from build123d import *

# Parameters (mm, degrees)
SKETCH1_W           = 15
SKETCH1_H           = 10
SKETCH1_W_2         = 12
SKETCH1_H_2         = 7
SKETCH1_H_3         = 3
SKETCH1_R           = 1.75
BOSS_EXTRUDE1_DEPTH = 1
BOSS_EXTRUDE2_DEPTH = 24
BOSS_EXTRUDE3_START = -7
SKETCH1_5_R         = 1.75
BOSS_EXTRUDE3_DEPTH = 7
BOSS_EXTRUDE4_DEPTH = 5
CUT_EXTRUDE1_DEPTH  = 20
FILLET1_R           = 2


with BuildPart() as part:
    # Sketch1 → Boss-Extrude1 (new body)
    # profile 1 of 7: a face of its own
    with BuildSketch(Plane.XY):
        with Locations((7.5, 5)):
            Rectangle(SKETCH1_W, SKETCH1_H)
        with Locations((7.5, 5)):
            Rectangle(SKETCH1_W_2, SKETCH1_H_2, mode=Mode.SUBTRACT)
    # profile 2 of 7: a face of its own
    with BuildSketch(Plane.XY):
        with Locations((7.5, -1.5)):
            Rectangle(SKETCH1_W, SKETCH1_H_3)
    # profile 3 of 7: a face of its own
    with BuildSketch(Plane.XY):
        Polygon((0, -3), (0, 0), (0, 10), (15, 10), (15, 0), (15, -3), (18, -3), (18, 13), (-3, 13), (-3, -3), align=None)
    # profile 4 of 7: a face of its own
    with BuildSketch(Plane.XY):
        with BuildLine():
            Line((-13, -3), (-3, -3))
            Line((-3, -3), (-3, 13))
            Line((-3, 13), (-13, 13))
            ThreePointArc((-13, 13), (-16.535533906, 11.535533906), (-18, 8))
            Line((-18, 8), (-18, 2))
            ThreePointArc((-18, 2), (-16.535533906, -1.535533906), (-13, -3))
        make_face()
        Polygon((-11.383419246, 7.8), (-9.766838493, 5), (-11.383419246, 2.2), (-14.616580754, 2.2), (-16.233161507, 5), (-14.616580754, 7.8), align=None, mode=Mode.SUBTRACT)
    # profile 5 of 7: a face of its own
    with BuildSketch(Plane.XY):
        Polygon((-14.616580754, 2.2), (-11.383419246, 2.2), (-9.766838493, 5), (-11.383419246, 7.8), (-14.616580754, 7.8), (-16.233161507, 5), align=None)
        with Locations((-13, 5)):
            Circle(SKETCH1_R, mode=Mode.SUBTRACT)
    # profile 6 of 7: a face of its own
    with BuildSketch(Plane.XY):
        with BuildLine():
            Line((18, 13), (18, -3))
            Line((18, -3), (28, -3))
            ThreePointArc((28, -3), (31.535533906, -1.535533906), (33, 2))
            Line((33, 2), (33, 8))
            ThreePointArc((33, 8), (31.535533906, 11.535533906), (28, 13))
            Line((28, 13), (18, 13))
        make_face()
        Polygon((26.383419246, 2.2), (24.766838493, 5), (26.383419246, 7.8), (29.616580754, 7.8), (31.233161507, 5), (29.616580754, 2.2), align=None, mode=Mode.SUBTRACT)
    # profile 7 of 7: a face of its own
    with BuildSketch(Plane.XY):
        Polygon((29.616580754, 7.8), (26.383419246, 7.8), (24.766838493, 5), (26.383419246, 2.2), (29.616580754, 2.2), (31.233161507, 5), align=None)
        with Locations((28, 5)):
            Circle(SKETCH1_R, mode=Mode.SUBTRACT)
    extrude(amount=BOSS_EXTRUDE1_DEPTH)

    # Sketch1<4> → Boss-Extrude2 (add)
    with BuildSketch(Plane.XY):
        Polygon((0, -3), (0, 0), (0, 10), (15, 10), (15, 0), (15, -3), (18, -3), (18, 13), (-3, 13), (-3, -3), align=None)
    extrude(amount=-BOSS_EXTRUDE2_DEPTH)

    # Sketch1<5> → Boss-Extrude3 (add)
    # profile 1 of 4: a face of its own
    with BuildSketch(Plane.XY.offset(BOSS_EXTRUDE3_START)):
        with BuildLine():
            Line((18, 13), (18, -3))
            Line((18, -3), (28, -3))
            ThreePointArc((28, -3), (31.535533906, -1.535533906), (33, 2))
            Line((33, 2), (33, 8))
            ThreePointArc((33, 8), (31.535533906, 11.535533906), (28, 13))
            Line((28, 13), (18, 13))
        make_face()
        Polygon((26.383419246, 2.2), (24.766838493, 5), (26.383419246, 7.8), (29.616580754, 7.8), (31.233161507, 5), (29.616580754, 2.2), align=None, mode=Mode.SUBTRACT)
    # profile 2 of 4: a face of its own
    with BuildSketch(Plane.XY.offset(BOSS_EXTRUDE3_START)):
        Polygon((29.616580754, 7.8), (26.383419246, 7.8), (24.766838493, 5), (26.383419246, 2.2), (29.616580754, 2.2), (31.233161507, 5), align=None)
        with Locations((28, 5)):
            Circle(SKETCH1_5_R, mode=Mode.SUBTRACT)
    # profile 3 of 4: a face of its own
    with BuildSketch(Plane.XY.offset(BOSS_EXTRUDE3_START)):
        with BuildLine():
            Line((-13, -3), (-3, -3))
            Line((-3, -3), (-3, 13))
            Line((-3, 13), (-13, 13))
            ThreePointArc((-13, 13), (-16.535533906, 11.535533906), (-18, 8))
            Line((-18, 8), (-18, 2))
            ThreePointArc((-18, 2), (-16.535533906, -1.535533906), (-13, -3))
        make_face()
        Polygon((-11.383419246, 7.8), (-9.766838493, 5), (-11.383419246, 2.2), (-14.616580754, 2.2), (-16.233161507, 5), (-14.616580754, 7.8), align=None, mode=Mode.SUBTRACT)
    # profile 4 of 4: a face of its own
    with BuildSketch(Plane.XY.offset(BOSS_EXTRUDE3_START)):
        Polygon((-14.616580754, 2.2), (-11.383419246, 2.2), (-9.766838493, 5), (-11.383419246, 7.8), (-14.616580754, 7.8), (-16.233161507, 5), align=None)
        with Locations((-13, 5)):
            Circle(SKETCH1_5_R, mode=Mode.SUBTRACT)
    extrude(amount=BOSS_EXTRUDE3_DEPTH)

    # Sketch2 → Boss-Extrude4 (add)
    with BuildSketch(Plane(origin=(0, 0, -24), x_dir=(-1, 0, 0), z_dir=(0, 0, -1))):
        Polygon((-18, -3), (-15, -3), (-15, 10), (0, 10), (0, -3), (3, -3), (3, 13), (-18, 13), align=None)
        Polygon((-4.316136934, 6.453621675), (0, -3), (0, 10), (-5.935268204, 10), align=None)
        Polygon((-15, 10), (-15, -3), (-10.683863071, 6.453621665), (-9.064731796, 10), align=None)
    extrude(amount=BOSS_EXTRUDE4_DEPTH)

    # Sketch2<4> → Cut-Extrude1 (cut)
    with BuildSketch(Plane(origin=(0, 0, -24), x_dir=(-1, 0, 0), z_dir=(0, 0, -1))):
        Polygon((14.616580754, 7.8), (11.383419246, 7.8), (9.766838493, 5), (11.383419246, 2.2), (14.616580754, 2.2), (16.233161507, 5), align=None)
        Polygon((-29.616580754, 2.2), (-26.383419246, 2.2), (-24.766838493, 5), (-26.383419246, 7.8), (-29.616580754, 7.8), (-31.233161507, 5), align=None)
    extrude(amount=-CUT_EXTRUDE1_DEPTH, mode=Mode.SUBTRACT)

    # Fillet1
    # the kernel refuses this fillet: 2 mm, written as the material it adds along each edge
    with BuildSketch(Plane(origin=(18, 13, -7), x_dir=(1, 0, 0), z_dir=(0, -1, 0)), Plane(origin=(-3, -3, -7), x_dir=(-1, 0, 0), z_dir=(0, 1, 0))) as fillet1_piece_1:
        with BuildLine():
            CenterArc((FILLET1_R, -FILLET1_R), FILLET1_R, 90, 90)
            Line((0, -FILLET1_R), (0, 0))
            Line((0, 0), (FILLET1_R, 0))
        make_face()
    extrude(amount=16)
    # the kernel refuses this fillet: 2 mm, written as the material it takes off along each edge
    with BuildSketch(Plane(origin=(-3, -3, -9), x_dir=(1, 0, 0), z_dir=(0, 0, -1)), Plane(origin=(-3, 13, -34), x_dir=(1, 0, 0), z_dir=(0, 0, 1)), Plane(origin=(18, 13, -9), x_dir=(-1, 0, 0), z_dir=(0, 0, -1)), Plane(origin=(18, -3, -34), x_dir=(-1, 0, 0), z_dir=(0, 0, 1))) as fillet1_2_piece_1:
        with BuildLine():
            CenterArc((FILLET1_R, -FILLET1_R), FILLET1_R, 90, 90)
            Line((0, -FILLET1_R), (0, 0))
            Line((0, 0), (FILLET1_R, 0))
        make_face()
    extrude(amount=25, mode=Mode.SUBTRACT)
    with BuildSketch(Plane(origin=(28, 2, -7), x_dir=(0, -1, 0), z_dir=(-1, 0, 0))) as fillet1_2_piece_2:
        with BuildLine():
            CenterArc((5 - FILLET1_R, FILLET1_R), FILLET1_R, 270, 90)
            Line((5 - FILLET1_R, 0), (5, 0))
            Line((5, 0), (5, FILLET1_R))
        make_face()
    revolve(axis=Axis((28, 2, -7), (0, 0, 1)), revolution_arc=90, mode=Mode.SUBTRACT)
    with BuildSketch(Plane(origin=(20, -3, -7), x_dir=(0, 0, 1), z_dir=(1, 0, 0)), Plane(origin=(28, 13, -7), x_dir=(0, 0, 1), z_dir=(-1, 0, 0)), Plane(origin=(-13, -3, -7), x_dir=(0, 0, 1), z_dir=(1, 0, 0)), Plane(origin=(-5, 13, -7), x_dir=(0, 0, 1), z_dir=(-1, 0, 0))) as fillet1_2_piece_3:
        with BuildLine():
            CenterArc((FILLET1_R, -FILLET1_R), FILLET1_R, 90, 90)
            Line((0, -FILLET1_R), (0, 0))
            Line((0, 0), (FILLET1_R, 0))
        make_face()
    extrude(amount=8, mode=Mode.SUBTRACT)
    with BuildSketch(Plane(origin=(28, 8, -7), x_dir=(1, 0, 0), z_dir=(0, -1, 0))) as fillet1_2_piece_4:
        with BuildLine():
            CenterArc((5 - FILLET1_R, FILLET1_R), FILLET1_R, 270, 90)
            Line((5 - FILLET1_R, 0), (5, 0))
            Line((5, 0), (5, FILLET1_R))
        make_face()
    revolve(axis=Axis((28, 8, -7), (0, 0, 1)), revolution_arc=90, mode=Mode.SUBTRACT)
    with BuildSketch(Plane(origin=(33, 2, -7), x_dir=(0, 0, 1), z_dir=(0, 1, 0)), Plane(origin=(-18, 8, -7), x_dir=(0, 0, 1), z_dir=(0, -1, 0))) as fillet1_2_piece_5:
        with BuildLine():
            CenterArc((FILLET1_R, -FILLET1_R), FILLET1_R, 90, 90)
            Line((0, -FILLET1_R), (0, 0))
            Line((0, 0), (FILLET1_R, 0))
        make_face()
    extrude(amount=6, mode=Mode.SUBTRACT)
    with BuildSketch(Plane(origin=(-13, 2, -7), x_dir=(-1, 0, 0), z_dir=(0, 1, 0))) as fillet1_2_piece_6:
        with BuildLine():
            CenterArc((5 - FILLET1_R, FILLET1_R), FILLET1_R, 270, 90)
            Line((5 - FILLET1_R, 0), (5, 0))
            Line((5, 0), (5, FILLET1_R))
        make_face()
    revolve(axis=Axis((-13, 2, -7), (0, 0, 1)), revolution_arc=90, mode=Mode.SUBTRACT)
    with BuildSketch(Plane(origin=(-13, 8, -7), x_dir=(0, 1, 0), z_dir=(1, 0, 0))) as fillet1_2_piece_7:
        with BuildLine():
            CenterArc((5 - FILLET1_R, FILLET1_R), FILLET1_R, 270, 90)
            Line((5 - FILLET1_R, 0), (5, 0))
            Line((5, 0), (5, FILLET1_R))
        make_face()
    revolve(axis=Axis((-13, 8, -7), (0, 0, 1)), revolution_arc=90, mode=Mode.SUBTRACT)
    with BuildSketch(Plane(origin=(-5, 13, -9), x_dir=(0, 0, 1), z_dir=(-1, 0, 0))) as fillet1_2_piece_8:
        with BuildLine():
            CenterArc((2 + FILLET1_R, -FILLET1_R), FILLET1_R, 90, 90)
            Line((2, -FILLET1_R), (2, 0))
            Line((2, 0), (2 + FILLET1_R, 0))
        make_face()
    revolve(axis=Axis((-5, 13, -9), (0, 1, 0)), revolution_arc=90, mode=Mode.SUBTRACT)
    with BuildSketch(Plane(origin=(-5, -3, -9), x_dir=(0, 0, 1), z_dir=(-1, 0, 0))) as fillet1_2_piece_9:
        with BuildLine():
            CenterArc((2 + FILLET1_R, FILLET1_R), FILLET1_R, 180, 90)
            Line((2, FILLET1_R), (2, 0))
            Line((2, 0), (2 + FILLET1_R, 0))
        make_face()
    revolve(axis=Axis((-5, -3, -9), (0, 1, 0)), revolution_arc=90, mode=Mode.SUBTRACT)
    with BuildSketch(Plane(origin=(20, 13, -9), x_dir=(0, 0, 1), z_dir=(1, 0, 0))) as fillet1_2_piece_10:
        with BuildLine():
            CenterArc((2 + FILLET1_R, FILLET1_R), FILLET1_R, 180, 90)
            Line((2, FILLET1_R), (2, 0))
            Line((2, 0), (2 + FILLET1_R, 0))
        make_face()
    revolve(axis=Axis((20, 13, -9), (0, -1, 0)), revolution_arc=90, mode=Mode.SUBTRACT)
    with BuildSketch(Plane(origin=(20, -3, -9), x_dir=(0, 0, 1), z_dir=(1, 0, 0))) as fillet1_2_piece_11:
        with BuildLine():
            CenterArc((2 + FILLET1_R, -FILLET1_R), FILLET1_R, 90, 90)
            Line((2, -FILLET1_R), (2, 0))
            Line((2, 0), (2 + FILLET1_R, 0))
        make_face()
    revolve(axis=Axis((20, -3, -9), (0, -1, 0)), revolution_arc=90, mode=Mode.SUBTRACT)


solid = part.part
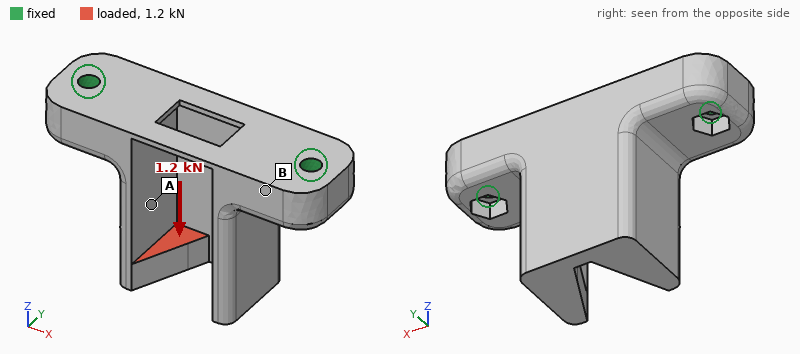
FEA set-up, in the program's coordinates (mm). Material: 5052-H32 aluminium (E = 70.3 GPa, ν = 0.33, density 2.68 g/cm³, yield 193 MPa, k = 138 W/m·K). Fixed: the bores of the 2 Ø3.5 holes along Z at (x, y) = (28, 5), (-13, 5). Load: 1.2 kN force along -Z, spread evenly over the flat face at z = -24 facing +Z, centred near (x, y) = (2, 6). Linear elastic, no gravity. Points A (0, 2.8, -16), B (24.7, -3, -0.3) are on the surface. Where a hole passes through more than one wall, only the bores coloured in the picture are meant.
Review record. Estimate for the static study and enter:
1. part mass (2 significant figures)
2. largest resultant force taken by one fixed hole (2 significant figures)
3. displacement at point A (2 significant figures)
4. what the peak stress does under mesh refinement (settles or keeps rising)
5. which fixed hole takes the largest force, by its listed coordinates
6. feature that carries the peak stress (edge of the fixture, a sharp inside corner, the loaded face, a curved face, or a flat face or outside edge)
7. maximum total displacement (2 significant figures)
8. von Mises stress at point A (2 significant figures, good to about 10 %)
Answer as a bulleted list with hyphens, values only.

- 21 g
- 860 N
- 22 µm
- keeps rising
- (-13, 5)
- edge of the fixture
- 43 µm
- 24 MPa
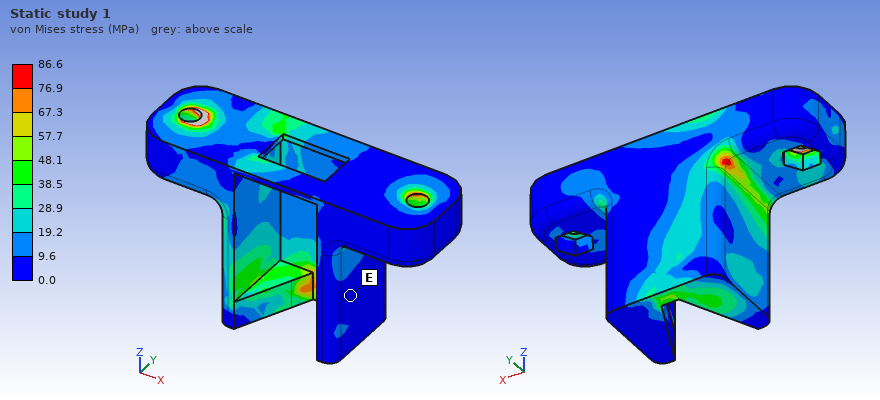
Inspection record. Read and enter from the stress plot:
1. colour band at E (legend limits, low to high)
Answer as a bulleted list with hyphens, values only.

- 0.0 to 9.6 MPa
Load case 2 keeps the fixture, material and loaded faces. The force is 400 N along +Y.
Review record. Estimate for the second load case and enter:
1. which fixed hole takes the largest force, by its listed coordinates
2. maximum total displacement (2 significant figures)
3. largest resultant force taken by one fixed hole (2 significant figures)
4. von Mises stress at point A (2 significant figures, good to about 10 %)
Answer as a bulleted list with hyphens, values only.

- (-13, 5)
- 72 µm
- 280 N
- 13 MPa
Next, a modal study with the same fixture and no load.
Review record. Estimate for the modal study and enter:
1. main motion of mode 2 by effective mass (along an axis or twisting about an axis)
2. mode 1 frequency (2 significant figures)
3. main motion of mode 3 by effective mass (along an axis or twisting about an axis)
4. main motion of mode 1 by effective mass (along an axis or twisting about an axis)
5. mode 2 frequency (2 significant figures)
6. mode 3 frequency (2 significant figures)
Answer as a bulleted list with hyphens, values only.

- along X
- 5600 Hz
- along Z
- along Y
- 7500 Hz
- 12 kHz
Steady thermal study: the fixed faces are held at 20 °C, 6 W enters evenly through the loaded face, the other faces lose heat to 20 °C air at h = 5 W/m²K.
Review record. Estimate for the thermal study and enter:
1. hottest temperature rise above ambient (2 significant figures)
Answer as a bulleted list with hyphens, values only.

- 15 K
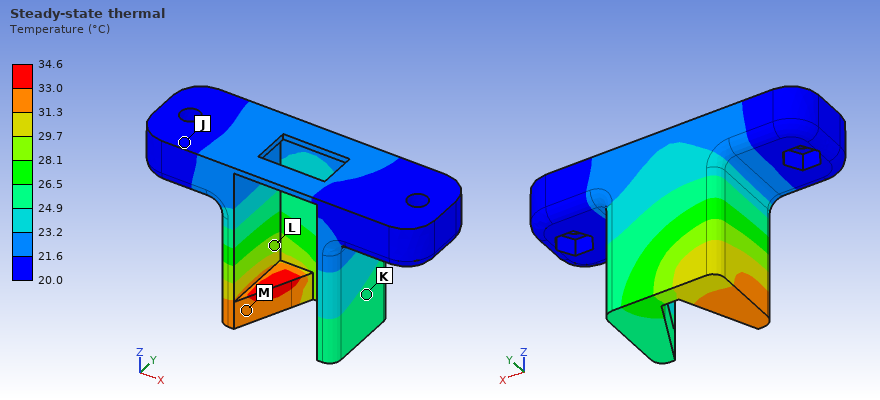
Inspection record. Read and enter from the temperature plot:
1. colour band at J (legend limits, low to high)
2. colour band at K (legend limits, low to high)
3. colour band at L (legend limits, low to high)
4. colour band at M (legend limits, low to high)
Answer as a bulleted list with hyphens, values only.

- 20.0 to 21.6 °C
- 24.9 to 26.5 °C
- 28.1 to 29.7 °C
- 31.3 to 33.0 °C
